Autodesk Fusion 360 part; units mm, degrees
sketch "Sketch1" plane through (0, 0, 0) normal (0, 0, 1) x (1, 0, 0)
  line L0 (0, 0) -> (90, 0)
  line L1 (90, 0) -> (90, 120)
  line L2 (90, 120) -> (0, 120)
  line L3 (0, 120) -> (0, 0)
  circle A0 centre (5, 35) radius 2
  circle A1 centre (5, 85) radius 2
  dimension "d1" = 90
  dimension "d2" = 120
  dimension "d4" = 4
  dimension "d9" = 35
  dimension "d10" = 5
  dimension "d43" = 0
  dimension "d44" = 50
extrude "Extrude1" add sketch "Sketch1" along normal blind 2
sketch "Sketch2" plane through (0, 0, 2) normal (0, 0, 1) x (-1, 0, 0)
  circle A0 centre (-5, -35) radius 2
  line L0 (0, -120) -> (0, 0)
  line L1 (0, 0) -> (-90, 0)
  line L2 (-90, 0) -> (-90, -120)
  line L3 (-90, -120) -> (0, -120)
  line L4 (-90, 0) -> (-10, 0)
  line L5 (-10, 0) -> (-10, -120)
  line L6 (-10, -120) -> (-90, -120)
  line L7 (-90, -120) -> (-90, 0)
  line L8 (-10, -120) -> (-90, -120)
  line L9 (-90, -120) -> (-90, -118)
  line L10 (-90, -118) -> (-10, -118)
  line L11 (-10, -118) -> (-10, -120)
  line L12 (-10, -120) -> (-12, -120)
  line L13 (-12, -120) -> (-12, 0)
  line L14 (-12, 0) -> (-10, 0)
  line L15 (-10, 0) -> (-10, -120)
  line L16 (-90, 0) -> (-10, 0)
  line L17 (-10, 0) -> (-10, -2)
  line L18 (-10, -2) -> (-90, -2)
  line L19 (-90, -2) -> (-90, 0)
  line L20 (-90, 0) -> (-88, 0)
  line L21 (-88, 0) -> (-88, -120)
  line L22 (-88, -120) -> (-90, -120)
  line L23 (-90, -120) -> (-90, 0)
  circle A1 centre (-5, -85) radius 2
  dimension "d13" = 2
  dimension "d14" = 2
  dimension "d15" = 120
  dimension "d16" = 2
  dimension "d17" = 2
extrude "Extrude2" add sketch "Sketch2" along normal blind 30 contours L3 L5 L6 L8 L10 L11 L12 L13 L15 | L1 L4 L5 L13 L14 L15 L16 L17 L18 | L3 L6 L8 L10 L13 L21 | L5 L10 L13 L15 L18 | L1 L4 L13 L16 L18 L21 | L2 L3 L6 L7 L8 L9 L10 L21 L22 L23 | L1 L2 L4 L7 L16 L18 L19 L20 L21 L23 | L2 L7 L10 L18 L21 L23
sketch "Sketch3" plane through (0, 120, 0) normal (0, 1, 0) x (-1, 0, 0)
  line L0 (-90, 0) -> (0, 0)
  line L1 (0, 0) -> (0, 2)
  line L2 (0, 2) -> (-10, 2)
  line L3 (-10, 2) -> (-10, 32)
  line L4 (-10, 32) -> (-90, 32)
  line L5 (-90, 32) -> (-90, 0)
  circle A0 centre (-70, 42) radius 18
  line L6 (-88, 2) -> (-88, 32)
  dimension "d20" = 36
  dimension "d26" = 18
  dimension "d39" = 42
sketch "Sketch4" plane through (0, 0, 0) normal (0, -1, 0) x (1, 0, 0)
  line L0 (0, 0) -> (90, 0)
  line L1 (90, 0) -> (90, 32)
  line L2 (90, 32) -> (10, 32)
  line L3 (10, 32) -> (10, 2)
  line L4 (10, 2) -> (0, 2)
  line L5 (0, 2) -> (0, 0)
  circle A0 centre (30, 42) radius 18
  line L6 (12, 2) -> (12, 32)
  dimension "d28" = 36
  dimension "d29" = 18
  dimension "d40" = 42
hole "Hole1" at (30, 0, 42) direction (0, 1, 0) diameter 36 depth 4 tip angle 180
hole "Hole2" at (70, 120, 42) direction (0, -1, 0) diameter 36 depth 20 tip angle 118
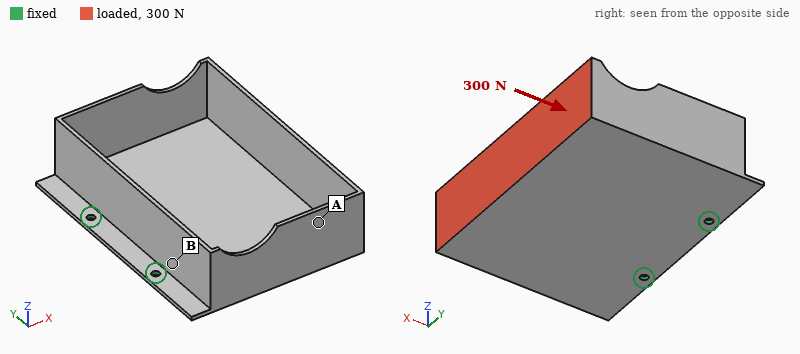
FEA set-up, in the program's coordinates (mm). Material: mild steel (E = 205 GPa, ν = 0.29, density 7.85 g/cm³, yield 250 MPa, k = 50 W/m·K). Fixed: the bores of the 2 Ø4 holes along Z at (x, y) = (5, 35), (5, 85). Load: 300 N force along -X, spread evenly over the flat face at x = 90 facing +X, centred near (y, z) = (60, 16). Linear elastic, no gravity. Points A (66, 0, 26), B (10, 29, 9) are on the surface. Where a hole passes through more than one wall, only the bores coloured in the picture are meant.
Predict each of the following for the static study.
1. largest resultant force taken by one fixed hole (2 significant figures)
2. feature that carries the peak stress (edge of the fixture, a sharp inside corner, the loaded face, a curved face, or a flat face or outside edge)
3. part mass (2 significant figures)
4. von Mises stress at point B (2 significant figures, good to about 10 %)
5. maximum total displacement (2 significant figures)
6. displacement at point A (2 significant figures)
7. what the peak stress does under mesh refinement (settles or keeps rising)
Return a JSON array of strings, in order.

["160 N", "edge of the fixture", "350 g", "23 MPa", "0.59 mm", "0.39 mm", "keeps rising"]
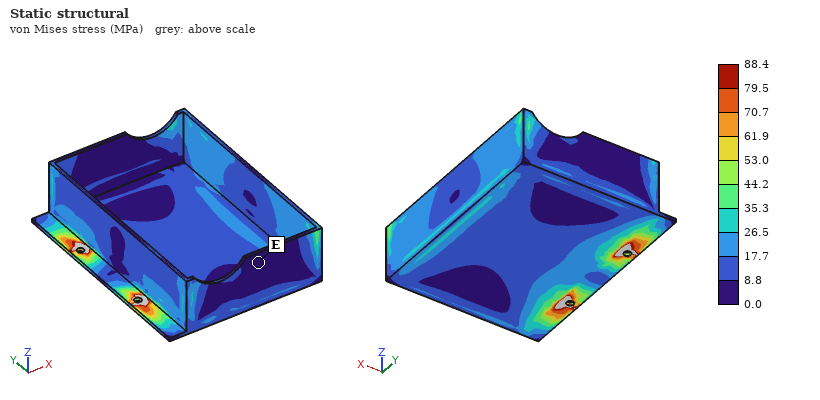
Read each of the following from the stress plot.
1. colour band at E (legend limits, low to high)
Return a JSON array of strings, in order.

["0.0 to 8.8 MPa"]
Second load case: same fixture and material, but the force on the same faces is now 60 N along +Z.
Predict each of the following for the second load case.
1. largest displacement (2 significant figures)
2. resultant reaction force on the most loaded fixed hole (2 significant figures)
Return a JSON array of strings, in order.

["0.56 mm", "31 N"]
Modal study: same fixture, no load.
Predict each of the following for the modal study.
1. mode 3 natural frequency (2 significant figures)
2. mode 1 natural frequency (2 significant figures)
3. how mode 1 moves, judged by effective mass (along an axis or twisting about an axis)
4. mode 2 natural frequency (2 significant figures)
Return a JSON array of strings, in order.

["1300 Hz", "150 Hz", "along Z", "320 Hz"]
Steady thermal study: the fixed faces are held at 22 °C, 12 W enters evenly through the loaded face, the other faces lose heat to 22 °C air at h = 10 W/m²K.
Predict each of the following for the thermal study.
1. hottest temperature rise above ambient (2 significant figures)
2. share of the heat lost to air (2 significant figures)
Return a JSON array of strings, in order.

["50 K", "69 %"]
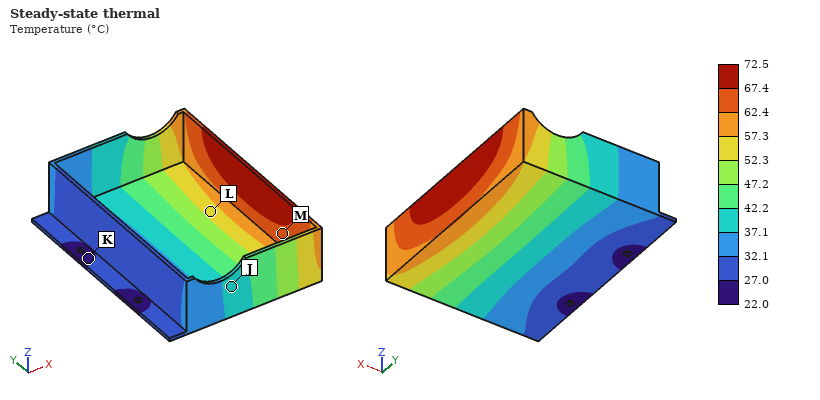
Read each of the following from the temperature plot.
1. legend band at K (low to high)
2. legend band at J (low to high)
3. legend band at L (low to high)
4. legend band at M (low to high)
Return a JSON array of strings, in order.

["22.0 to 27.0 °C", "37.1 to 42.2 °C", "52.3 to 57.3 °C", "62.4 to 67.4 °C"]
